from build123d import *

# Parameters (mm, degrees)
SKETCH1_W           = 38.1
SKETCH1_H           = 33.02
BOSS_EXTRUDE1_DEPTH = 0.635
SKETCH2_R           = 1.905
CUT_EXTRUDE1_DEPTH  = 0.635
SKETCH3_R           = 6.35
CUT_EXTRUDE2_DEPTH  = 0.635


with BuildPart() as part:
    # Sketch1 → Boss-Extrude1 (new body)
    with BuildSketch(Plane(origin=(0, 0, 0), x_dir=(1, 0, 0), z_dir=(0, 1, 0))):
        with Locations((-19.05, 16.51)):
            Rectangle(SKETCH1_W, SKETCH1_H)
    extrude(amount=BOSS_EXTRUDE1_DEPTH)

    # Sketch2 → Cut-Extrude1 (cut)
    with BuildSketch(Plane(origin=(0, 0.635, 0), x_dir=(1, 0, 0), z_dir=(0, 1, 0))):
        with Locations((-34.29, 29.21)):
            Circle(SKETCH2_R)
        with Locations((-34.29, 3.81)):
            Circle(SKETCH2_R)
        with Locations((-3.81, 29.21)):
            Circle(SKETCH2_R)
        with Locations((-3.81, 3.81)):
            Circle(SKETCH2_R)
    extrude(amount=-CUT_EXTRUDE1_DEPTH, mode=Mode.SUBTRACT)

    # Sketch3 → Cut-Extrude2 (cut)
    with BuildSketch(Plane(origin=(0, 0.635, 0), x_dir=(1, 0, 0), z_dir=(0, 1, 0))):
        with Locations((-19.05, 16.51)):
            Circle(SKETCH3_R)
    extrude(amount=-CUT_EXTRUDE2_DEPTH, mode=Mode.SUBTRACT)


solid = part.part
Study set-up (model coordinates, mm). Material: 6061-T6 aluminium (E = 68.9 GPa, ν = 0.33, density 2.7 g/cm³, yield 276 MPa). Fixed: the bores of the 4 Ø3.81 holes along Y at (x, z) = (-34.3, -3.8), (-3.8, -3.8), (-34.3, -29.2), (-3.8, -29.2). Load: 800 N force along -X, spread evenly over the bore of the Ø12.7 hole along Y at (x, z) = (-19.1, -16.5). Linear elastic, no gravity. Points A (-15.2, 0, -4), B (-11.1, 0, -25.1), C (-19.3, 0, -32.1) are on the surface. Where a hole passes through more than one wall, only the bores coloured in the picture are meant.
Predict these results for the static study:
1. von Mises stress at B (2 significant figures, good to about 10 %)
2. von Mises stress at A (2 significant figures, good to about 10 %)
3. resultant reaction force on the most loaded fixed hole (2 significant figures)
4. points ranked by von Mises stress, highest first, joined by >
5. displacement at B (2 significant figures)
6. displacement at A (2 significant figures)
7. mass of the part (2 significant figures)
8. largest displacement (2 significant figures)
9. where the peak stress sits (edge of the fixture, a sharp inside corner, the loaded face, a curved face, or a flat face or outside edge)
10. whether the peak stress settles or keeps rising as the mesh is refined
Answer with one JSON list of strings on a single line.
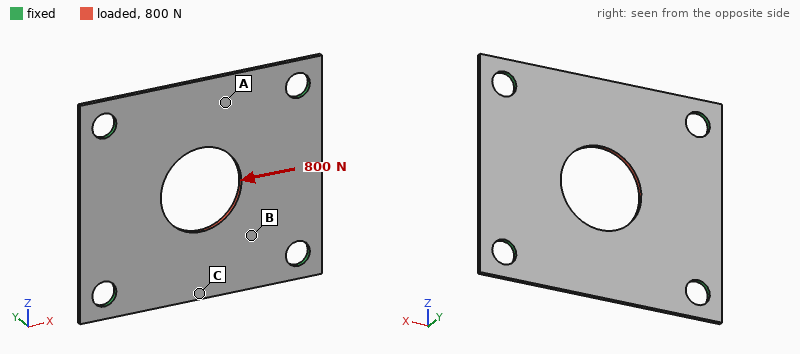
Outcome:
["32 MPa", "16 MPa", "220 N", "B > A > C", "4.2 µm", "3.2 µm", "1.9 g", "9.2 µm", "edge of the fixture", "keeps rising"]
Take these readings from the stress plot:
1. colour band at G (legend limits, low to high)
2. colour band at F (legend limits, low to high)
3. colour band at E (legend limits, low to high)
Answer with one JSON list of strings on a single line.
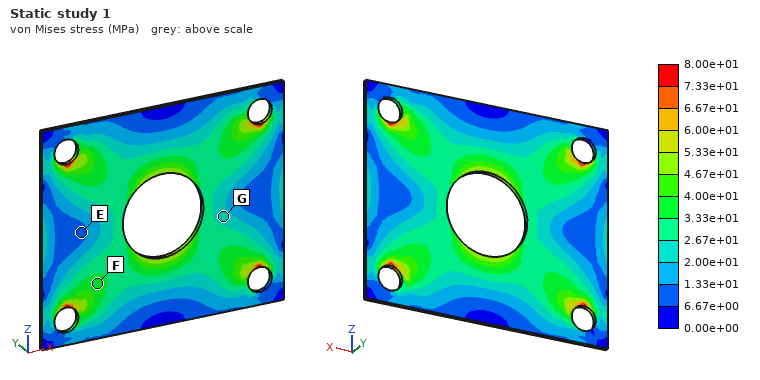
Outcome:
["2.00e+01 to 2.67e+01 MPa", "3.33e+01 to 4.00e+01 MPa", "6.67e+00 to 1.33e+01 MPa"]
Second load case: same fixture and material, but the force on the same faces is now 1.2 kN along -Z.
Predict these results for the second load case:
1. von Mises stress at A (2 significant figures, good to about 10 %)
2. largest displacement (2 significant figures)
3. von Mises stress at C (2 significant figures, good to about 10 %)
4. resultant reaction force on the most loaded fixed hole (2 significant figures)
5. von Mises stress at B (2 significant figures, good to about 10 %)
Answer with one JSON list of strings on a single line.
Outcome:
["31 MPa", "19 µm", "43 MPa", "340 N", "54 MPa"]
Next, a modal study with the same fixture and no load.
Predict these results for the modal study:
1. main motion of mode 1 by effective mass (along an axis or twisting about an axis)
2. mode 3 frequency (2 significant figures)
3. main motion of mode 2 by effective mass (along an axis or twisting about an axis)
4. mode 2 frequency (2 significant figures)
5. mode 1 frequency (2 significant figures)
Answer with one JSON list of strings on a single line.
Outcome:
["along Y", "5900 Hz", "twisting about X", "4800 Hz", "3800 Hz"]
